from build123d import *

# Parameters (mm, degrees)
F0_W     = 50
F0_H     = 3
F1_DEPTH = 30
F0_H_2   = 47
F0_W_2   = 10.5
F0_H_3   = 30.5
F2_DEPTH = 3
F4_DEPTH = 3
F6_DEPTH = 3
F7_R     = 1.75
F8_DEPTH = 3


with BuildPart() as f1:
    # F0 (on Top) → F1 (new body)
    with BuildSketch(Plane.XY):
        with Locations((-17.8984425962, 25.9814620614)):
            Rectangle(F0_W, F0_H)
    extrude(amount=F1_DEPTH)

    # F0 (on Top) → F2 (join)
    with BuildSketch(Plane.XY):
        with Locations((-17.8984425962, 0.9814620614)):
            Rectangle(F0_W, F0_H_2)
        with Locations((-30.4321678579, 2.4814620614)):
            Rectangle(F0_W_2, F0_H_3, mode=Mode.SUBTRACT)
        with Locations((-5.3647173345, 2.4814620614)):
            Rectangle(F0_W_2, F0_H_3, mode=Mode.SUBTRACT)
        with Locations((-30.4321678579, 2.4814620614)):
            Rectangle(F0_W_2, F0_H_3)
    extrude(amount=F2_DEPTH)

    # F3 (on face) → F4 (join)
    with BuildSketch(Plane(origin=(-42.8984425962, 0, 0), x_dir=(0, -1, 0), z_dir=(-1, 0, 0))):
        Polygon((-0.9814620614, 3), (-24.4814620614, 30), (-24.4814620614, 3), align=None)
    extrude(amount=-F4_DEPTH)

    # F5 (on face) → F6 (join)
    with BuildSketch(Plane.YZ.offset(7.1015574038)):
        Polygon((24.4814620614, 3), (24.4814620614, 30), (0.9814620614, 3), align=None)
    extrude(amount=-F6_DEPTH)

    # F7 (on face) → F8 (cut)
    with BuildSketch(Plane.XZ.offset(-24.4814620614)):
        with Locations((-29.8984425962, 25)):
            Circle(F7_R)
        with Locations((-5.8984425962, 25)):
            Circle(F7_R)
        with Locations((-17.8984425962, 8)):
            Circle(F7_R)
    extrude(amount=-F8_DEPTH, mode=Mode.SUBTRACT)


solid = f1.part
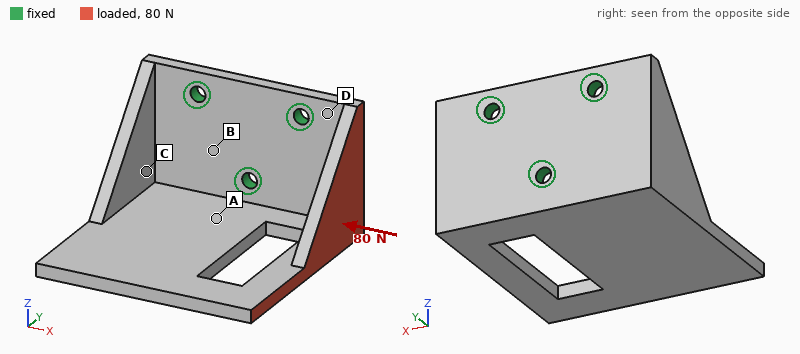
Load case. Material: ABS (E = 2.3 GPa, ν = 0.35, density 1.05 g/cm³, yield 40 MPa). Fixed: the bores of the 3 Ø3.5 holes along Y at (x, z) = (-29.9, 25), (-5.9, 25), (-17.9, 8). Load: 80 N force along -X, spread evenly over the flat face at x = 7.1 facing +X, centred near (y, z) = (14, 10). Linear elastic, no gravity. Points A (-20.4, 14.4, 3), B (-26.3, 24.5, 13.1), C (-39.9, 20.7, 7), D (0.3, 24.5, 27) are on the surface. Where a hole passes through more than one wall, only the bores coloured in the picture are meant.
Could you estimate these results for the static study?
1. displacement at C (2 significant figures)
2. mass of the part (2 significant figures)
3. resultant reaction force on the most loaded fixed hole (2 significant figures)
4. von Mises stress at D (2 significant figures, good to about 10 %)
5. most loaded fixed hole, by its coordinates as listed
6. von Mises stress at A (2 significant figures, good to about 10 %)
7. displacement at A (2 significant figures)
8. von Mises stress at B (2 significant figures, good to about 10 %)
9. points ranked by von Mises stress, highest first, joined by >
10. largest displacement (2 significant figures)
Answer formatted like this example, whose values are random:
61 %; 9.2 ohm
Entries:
0.25 mm; 13 g; 55 N; 6.6 MPa; (-17.9, 8); 2.0 MPa; 0.17 mm; 4.1 MPa; D > B > A > C; 0.87 mm
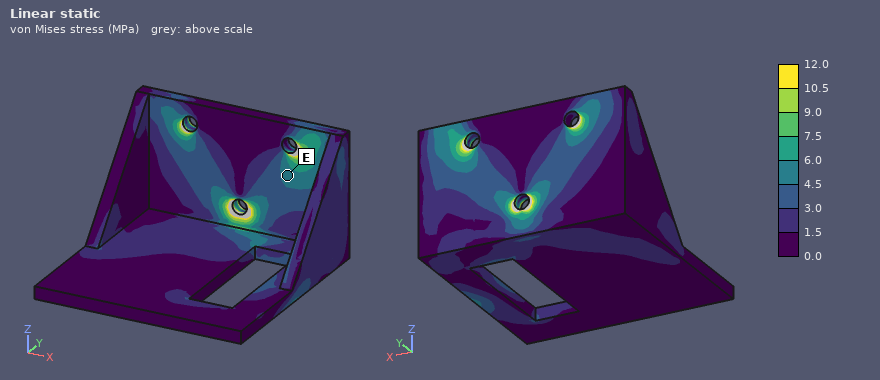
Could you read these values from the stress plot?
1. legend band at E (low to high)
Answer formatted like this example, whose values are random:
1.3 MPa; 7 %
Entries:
4.5 to 6.0 MPa
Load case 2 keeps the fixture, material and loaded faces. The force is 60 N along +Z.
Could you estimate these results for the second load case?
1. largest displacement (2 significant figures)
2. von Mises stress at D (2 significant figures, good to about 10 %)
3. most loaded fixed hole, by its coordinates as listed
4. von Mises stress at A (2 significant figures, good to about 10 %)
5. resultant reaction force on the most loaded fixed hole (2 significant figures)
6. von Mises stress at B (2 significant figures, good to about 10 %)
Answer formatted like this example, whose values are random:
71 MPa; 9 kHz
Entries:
0.91 mm; 5.1 MPa; (-5.9, 25); 1.7 MPa; 71 N; 1.6 MPa
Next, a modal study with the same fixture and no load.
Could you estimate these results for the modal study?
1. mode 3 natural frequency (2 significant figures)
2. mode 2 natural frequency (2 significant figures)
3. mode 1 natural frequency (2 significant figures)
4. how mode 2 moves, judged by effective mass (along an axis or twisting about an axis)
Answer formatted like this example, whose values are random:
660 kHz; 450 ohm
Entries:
1200 Hz; 490 Hz; 440 Hz; along Z
